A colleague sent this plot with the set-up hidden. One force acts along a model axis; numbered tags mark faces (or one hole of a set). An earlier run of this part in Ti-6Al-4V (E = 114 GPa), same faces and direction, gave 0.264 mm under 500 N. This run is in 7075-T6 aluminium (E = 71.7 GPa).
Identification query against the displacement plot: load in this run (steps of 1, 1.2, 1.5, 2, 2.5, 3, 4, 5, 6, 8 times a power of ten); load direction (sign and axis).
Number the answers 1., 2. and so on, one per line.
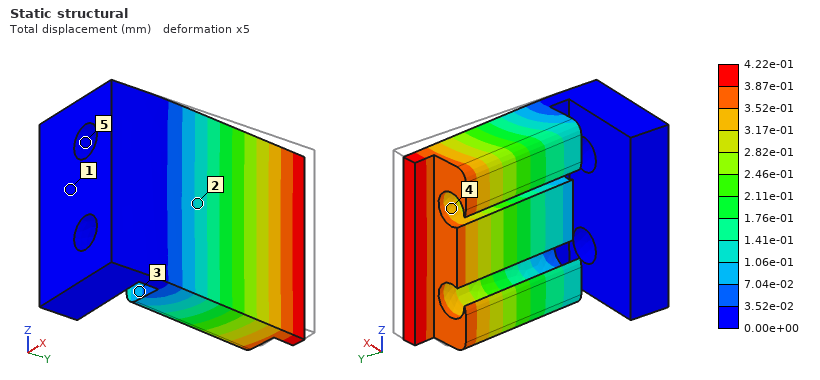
1. 500 N
2. -X
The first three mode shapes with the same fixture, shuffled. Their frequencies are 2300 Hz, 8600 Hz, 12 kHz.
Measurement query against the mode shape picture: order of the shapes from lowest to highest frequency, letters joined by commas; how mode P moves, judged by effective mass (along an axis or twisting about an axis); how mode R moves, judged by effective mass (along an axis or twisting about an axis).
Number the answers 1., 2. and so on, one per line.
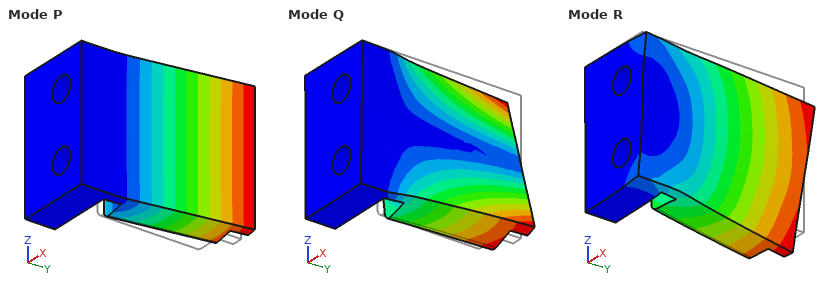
1. P, Q, R
2. along X
3. along Z
